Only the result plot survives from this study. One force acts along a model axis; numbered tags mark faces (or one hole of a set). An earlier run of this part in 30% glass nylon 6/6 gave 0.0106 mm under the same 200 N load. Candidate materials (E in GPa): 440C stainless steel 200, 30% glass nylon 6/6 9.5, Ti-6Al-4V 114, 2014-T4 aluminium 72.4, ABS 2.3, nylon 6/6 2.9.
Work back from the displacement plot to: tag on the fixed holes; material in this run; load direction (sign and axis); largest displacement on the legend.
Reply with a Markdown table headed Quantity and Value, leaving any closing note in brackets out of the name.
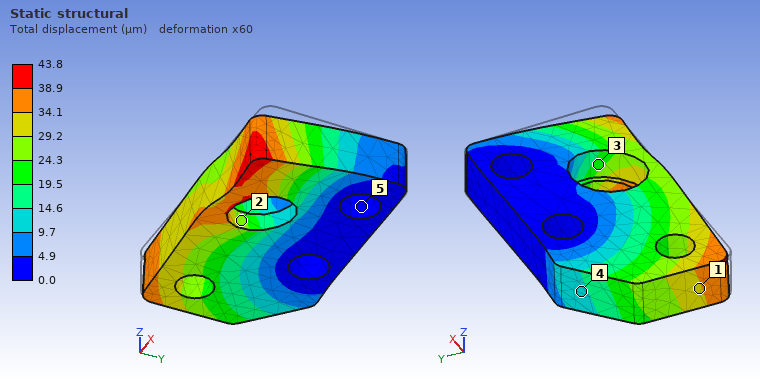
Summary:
| Quantity | Value |
|---|---|
| tag on the fixed holes | 5 |
| material in this run | ABS |
| load direction | -X |
| largest displacement on the legend | 43.8 µm |
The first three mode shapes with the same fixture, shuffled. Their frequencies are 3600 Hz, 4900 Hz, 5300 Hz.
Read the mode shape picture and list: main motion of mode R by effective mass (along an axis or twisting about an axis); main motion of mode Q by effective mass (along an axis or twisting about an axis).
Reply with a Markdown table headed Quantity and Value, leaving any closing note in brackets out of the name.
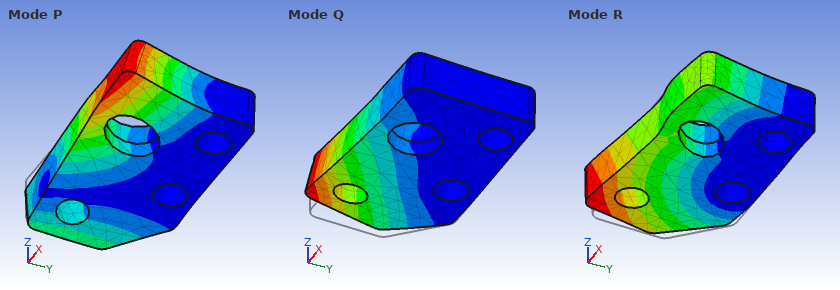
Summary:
| Quantity | Value |
|---|---|
| main motion of mode R by effective mass | along X |
| main motion of mode Q by effective mass | along Z |
